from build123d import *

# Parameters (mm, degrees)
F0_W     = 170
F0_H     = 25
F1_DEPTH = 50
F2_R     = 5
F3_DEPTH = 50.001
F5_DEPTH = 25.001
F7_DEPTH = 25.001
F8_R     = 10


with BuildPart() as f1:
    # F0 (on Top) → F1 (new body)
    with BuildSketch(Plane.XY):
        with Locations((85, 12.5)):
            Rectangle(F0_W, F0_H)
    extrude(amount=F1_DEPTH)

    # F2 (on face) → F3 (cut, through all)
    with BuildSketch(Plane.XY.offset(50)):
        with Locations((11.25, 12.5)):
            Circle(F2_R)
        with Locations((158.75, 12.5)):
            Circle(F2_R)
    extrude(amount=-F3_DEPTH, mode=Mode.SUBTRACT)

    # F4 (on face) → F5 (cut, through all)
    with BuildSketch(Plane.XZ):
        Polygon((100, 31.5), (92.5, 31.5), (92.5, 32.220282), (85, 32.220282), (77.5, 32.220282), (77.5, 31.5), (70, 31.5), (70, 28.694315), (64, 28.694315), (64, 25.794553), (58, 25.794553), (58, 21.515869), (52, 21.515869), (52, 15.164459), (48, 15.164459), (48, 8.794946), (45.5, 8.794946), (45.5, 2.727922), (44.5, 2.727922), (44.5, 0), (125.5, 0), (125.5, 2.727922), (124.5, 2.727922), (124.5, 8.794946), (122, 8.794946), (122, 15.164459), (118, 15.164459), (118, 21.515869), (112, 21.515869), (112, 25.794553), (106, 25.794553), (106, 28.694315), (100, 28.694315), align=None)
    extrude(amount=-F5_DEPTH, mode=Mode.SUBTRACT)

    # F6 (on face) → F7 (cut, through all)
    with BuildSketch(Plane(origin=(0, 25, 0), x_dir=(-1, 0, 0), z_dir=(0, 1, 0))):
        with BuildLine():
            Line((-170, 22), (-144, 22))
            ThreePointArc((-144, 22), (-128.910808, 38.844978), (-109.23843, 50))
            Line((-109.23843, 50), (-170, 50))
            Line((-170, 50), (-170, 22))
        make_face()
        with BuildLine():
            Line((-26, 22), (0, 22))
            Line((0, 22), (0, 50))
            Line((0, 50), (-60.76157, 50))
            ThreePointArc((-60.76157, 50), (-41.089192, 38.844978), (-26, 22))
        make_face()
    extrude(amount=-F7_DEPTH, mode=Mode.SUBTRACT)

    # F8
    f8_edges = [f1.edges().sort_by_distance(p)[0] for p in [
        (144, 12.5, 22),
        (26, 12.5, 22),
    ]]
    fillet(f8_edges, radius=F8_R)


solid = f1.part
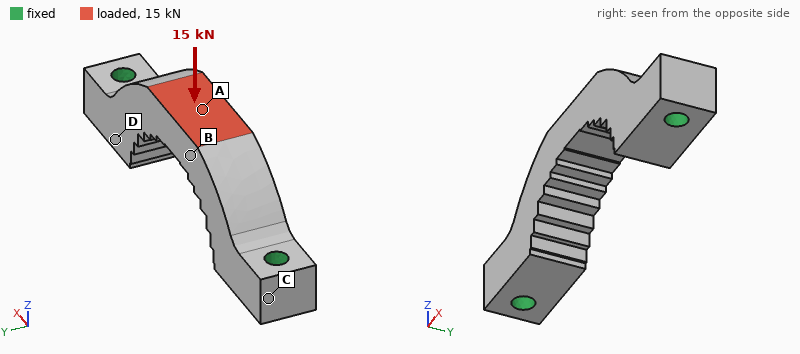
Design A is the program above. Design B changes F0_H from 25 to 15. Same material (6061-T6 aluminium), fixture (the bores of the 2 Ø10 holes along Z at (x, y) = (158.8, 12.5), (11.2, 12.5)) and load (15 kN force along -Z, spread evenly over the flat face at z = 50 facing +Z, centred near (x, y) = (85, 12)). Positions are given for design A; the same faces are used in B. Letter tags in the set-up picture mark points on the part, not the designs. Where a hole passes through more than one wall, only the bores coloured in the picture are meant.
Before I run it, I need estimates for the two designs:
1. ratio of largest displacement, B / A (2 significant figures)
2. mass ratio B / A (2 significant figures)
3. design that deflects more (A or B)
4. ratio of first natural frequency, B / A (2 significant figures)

1.6
0.59
B
0.77
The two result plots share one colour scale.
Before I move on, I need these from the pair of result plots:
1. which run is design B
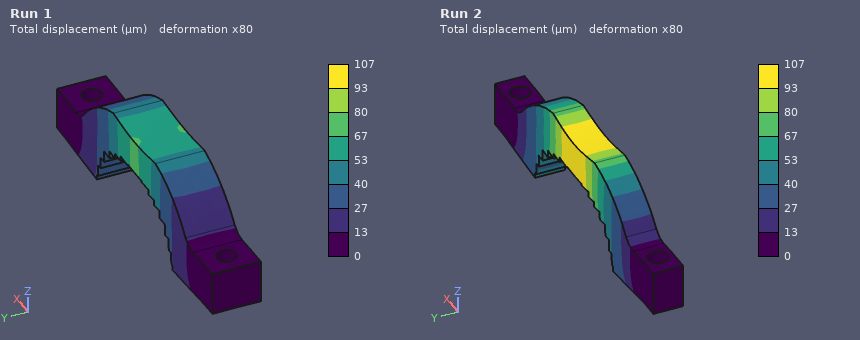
Run 2
